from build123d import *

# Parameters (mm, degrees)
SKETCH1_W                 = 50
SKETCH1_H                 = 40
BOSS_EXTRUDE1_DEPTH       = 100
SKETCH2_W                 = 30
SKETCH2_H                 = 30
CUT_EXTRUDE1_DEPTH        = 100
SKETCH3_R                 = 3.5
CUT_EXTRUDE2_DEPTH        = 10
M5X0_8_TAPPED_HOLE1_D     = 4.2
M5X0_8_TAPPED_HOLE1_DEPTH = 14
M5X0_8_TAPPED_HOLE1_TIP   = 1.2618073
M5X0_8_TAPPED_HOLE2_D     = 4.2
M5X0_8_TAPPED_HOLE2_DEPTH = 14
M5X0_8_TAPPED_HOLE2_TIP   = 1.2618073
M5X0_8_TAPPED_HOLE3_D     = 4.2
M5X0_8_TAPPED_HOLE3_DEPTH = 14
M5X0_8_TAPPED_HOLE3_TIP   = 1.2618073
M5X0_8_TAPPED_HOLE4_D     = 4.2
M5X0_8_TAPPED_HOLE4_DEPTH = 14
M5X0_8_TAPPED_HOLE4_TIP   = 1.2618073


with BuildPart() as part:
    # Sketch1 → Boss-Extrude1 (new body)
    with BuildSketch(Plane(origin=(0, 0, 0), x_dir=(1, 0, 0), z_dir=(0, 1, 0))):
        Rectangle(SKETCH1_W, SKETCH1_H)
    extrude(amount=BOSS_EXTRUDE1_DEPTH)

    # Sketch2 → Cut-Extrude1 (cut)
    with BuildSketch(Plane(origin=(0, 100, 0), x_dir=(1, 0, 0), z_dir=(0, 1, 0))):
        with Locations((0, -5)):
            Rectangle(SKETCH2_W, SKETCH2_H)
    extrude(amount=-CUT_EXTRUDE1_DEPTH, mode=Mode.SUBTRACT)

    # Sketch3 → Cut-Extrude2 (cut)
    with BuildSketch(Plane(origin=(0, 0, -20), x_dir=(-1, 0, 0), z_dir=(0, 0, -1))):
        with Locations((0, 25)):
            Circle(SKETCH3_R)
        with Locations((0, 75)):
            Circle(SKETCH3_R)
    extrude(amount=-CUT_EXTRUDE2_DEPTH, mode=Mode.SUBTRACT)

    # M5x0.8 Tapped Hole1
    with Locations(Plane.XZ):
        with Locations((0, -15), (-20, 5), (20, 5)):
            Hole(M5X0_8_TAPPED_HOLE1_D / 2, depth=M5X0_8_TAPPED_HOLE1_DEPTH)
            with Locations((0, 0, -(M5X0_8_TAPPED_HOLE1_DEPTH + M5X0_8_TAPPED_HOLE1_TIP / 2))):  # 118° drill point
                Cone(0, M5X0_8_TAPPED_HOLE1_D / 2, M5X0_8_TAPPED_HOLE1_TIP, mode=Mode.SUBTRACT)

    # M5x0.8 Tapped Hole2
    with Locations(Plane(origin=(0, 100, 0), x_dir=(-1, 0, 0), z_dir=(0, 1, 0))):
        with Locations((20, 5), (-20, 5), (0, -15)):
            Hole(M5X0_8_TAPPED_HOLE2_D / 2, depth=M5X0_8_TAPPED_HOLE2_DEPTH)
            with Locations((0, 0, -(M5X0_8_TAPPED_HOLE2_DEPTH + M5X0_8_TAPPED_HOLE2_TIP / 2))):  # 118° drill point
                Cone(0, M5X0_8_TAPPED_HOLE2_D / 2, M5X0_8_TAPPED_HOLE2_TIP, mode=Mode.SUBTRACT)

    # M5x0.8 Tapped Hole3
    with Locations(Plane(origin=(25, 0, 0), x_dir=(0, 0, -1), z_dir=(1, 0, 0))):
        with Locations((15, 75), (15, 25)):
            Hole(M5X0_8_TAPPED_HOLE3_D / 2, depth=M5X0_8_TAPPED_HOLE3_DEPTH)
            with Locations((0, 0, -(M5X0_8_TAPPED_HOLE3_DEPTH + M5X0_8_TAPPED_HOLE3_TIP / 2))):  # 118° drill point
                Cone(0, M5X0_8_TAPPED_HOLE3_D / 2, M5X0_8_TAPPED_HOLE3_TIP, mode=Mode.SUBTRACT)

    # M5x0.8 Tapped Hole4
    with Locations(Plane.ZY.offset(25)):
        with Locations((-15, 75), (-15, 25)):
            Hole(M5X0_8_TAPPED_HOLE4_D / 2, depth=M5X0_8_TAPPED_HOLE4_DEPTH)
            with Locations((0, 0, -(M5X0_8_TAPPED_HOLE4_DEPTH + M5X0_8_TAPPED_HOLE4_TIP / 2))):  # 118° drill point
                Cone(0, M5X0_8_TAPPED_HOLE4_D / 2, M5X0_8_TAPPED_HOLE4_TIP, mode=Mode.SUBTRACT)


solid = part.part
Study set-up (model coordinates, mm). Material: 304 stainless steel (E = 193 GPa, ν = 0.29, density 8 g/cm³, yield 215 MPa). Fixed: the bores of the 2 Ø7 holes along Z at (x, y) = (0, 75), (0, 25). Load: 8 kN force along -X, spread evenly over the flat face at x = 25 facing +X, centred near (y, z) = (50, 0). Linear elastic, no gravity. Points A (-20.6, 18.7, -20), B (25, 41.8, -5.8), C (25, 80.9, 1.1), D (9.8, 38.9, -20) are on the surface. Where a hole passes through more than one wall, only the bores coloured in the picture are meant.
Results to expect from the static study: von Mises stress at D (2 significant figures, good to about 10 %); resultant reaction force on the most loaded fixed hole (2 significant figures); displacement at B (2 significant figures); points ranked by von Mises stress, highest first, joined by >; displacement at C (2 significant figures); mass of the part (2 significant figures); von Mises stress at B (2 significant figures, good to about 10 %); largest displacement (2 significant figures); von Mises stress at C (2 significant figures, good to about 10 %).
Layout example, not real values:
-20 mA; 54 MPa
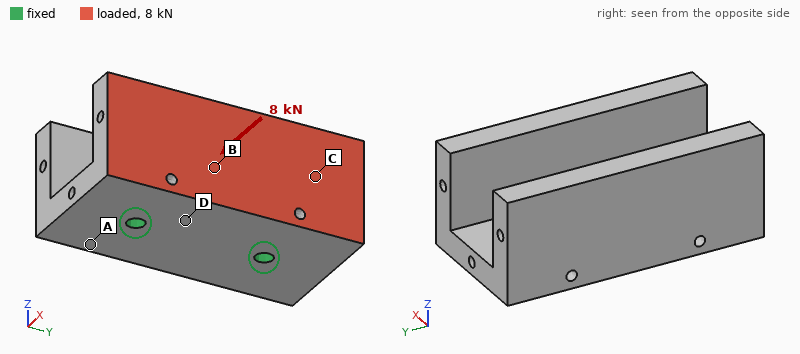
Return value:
53 MPa; 4.0 kN; 35 µm; D > B > C > A; 45 µm; 860 g; 39 MPa; 83 µm; 21 MPa
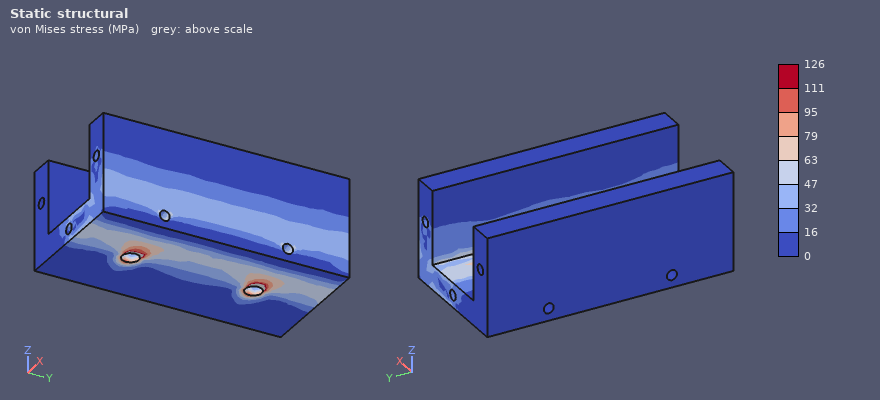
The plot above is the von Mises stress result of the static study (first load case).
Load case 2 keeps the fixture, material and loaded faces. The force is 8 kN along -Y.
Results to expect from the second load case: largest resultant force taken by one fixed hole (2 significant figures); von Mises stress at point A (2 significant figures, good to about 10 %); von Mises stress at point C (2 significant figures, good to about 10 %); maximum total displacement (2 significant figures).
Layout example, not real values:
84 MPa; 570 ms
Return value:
5.7 kN; 9.3 MPa; 9.9 MPa; 18 µm
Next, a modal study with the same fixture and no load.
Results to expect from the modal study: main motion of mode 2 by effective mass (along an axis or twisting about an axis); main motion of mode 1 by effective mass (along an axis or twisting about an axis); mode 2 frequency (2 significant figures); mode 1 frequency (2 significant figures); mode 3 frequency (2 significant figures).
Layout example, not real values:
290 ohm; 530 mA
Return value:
along Z; along X; 3500 Hz; 2700 Hz; 4300 Hz
